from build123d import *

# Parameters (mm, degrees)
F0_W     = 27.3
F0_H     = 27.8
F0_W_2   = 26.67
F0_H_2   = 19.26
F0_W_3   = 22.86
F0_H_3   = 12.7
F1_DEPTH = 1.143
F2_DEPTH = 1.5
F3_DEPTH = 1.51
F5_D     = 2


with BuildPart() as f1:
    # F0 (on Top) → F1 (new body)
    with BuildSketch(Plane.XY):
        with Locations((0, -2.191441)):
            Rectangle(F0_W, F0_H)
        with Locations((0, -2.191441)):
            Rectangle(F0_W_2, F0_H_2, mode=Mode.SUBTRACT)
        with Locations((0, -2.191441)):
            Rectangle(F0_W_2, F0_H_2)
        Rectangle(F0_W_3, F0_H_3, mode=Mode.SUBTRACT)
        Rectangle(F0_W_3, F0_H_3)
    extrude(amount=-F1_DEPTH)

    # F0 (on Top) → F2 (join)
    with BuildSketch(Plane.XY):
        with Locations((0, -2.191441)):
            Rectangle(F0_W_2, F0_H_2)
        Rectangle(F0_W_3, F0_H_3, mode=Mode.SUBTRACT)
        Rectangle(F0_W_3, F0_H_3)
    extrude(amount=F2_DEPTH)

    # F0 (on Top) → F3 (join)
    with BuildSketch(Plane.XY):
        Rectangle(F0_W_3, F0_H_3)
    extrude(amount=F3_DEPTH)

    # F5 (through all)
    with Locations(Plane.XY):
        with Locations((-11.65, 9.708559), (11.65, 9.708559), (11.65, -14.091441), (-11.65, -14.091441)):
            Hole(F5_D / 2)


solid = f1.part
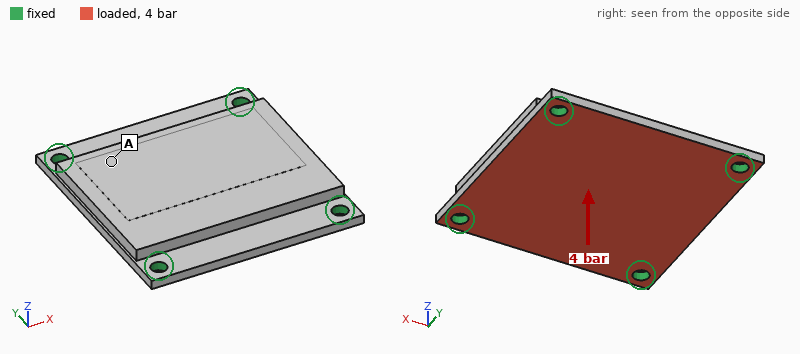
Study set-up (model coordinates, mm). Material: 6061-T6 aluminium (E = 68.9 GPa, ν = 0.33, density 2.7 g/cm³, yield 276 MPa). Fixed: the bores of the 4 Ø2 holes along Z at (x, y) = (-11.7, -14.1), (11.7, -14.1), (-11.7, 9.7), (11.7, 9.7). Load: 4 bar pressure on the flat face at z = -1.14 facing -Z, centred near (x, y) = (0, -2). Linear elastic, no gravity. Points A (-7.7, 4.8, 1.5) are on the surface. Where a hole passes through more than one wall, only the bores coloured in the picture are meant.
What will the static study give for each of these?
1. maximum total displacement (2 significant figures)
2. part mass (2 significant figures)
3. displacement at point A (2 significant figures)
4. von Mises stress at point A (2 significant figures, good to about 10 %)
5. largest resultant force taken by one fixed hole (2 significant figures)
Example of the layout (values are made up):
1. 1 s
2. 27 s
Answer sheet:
1. 16 µm
2. 4.4 g
3. 10.0 µm
4. 17 MPa
5. 110 N
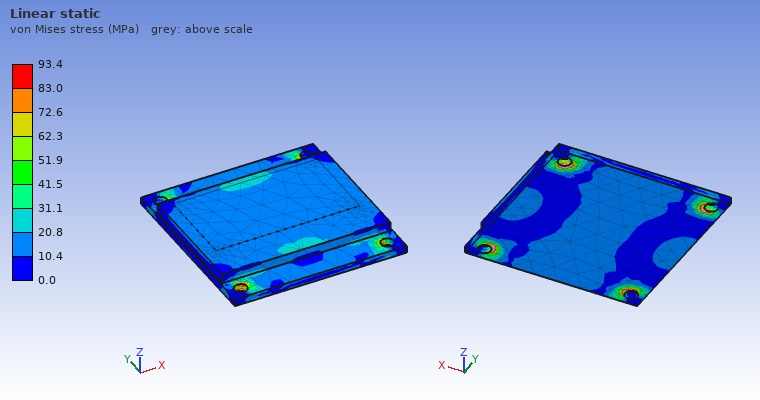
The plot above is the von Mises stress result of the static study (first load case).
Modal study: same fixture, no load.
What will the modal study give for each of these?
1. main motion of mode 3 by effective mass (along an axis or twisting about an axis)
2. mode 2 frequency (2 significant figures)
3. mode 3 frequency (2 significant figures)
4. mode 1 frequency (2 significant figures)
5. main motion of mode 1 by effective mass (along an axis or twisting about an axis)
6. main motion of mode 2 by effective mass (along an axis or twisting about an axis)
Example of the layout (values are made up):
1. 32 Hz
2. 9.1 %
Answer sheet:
1. twisting about Y
2. 19 kHz
3. 20 kHz
4. 11 kHz
5. along Z
6. twisting about X
